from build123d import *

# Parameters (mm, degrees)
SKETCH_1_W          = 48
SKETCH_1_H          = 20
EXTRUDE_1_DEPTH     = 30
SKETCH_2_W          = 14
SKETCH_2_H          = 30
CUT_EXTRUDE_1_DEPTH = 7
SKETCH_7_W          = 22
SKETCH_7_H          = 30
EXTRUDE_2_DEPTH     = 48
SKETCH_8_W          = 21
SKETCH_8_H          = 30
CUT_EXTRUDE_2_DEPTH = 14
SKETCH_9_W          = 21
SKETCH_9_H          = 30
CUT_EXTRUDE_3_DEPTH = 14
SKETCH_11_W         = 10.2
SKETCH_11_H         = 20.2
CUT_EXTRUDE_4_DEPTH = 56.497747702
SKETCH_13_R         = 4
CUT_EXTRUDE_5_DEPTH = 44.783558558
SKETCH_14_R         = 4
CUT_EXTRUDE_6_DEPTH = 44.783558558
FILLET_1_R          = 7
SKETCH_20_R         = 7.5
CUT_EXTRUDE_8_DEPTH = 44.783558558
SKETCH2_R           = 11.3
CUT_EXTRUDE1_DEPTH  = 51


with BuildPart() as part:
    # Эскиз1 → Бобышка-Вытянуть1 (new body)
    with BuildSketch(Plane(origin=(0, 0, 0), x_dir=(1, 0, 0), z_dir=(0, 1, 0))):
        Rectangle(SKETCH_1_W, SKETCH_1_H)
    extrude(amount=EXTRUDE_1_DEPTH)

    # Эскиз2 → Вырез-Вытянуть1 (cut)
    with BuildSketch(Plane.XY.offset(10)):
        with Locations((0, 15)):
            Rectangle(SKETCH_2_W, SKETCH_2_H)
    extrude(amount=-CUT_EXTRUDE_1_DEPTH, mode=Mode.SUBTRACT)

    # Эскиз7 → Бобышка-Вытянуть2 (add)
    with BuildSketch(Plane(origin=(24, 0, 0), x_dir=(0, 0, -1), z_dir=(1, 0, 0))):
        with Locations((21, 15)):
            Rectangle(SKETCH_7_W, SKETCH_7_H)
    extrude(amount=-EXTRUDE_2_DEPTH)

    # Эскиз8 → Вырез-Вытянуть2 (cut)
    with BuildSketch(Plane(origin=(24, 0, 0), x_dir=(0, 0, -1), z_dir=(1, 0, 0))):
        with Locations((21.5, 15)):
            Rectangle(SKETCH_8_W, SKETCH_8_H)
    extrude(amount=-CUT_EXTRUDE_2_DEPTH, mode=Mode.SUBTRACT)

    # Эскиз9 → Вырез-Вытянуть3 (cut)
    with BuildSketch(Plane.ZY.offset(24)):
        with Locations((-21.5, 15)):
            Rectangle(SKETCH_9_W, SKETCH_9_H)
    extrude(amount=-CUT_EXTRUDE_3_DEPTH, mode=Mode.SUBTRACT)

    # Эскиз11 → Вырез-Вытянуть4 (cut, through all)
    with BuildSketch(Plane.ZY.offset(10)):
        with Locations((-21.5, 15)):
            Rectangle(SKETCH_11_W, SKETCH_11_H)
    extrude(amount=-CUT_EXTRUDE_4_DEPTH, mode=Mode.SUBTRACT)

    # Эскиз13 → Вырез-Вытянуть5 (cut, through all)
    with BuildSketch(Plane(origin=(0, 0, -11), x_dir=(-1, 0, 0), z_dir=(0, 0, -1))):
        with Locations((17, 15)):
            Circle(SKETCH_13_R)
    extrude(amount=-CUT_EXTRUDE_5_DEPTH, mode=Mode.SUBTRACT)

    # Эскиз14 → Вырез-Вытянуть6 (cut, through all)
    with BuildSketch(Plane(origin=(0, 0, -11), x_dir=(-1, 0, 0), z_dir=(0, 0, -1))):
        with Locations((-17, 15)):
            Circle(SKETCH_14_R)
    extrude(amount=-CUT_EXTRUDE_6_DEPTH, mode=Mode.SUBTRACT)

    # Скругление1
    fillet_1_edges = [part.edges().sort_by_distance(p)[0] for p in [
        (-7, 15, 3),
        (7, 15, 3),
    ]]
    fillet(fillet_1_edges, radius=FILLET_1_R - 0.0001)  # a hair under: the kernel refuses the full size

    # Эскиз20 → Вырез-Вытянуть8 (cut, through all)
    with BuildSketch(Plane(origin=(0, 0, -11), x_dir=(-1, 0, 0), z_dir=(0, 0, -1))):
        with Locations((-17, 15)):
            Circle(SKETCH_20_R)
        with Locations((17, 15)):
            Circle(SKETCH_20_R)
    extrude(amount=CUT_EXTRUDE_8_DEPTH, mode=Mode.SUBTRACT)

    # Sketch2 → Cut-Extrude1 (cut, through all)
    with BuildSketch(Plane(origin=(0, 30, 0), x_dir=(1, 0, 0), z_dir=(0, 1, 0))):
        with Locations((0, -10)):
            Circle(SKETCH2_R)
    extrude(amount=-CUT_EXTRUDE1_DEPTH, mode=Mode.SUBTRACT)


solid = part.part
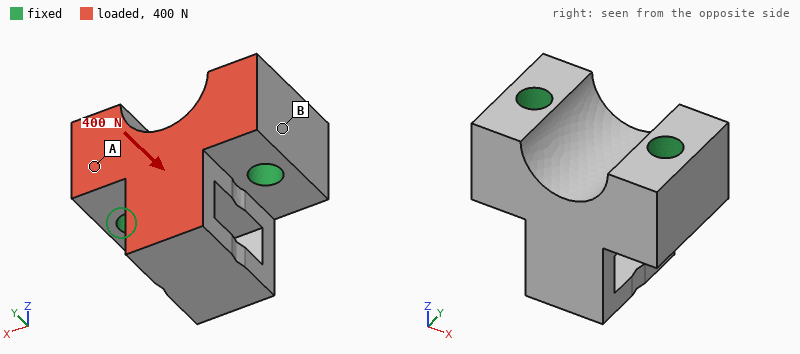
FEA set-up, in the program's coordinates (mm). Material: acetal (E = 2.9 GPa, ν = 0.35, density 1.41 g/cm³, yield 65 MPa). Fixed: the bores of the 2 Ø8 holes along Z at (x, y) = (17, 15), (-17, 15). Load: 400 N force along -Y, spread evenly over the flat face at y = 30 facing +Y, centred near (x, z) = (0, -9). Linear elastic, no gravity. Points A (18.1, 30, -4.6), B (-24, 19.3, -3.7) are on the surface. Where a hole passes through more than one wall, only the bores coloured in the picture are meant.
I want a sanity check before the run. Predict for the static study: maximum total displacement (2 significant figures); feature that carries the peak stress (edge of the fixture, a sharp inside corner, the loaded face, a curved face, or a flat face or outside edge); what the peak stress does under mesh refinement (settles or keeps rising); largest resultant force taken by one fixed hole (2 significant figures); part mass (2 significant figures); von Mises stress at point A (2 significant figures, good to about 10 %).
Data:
51 µm
edge of the fixture
keeps rising
200 N
43 g
0.57 MPa
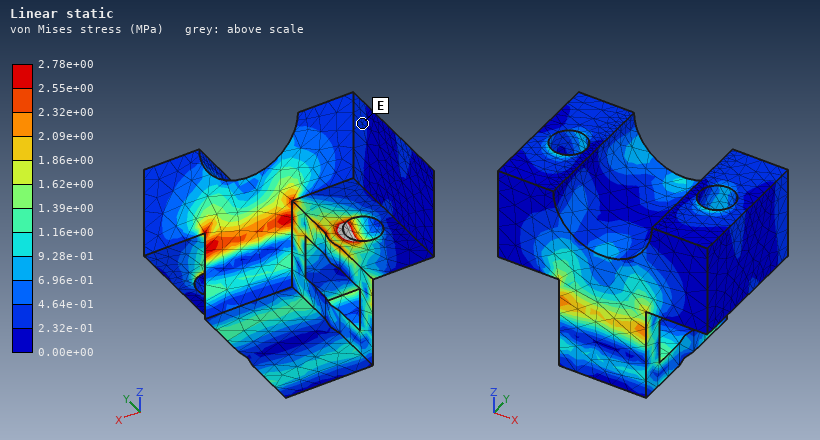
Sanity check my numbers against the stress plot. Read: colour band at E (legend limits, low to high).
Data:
2.32e-01 to 4.64e-01 MPa
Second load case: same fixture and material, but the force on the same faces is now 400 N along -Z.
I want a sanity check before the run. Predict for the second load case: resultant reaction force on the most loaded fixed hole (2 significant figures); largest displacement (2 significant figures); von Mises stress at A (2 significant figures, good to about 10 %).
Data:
210 N
40 µm
0.81 MPa
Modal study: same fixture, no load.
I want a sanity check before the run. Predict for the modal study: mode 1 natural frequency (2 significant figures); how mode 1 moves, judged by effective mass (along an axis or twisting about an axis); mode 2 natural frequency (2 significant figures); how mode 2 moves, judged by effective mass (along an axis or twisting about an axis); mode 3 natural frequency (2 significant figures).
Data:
2800 Hz
along Y
3900 Hz
along X
5700 Hz
